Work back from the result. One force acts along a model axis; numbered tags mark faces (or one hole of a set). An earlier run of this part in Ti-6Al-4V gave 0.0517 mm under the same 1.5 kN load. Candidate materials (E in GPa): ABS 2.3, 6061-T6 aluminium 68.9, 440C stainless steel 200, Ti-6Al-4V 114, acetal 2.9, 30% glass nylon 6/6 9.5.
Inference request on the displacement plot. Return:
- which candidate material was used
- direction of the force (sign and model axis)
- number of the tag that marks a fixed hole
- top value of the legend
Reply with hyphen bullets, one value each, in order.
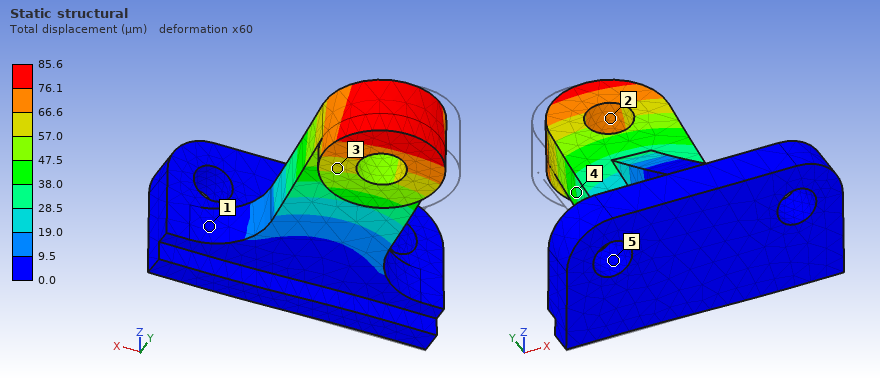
- 6061-T6 aluminium
- +X
- 5
- 85.6 µm
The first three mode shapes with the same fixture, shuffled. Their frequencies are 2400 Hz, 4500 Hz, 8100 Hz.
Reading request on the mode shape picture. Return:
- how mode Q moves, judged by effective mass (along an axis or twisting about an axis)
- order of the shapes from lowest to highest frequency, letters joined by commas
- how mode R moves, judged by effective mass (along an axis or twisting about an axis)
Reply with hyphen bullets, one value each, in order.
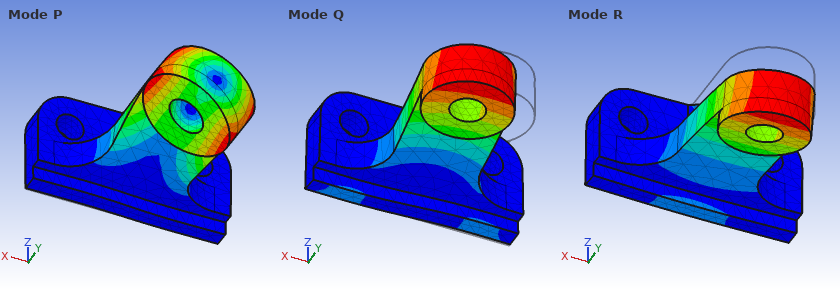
- along X
- R, Q, P
- along Z
